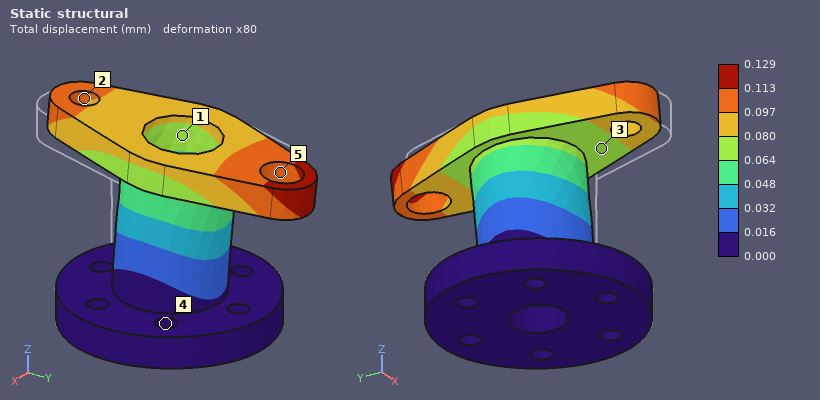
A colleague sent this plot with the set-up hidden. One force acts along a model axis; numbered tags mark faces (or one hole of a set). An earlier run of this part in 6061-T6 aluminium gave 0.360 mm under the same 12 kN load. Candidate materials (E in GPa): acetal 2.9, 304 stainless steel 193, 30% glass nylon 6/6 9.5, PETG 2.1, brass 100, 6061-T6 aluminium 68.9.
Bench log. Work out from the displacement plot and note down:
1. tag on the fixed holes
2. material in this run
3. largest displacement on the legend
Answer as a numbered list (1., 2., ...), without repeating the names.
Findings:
1. 4
2. 304 stainless steel
3. 0.129 mm
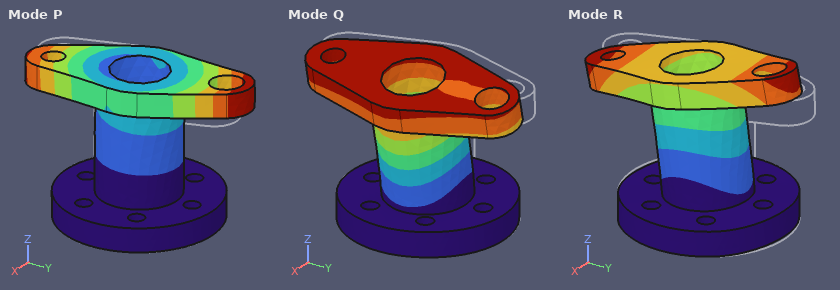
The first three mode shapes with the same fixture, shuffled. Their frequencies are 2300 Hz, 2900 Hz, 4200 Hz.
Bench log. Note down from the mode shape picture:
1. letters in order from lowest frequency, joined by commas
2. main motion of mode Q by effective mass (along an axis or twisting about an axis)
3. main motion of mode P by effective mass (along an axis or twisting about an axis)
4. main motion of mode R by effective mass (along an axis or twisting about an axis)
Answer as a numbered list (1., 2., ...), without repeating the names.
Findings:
1. R, Q, P
2. along X
3. twisting about Z
4. along Y
